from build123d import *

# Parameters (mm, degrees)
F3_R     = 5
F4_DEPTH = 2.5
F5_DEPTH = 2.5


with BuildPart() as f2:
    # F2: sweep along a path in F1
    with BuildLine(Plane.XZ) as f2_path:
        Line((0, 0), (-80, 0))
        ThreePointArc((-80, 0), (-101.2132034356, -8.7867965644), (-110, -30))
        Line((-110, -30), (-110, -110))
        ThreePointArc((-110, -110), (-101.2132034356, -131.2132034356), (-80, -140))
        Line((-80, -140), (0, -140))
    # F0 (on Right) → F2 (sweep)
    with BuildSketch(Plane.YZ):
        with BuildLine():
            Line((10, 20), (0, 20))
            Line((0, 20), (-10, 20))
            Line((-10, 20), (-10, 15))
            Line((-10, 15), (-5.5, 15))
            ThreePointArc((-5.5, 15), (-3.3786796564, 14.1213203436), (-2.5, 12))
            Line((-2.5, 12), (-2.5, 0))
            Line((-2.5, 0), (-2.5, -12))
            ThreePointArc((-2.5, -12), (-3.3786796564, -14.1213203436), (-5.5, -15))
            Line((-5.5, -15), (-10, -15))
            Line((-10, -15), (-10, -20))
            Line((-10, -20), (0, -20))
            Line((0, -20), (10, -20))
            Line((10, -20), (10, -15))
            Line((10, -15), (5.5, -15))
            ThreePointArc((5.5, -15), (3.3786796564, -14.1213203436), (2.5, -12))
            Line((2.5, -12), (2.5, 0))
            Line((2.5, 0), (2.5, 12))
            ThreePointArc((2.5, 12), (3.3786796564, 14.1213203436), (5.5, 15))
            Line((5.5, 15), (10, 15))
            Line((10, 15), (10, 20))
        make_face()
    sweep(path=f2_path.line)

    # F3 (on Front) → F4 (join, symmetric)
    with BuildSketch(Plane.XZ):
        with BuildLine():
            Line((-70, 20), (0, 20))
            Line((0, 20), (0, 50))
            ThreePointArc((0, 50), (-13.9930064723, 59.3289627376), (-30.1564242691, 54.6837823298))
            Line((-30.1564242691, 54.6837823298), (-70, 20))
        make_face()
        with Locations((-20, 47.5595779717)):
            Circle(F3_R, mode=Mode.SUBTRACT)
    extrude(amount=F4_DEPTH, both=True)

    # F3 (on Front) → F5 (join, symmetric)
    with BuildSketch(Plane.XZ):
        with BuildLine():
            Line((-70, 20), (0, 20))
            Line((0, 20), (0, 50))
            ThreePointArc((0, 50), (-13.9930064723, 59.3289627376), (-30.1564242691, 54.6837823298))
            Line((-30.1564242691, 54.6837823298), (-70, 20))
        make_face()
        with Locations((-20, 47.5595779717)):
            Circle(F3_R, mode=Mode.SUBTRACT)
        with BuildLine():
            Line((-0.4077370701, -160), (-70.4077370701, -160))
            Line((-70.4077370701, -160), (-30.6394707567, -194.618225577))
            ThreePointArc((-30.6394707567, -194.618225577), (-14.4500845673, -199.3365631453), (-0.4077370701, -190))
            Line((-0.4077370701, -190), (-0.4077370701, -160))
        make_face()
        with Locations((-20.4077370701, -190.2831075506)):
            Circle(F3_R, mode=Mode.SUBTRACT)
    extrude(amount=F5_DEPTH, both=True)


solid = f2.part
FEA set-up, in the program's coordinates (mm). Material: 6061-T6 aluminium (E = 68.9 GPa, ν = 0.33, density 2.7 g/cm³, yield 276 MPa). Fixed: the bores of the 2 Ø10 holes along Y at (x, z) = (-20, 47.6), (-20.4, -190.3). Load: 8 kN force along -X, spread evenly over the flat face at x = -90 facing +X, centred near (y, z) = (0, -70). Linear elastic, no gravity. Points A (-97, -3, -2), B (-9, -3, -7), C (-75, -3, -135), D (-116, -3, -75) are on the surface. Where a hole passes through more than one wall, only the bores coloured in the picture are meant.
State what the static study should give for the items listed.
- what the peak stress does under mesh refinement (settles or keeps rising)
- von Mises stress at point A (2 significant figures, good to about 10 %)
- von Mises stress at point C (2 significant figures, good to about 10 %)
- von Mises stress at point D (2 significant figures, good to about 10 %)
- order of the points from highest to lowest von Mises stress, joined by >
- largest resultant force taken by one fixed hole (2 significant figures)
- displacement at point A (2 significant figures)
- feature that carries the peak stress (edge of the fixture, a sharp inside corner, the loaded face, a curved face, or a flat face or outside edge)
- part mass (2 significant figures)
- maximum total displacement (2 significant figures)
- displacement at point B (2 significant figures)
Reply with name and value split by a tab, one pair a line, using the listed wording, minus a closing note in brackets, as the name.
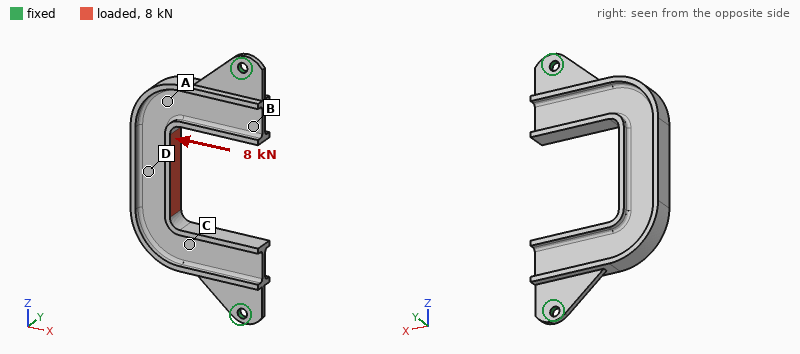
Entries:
what the peak stress does under mesh refinement	keeps rising
von Mises stress at point A	12 MPa
von Mises stress at point C	33 MPa
von Mises stress at point D	20 MPa
order of the points from highest to lowest von Mises stress, joined by >	C > D > A > B
largest resultant force taken by one fixed hole	5.1 kN
displacement at point A	0.045 mm
feature that carries the peak stress	edge of the fixture
part mass	370 g
maximum total displacement	0.11 mm
displacement at point B	0.044 mm
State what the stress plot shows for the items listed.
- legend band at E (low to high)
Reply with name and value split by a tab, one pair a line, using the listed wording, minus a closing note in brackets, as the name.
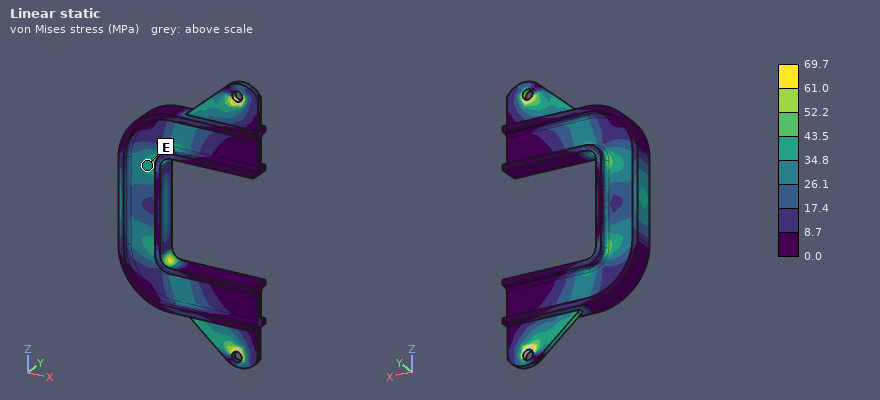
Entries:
legend band at E	34.8 to 43.5 MPa
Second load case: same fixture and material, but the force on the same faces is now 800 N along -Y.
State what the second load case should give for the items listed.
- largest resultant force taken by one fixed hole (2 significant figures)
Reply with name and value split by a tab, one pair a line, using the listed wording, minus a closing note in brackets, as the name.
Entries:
largest resultant force taken by one fixed hole	410 N
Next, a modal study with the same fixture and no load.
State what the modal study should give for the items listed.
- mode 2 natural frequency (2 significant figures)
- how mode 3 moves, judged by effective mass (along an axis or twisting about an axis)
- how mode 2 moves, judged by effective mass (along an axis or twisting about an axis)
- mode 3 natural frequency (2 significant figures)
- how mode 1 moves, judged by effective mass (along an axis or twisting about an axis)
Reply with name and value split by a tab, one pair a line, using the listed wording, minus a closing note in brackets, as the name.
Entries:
mode 2 natural frequency	720 Hz
how mode 3 moves, judged by effective mass	along Y
how mode 2 moves, judged by effective mass	twisting about X
mode 3 natural frequency	890 Hz
how mode 1 moves, judged by effective mass	along Y
